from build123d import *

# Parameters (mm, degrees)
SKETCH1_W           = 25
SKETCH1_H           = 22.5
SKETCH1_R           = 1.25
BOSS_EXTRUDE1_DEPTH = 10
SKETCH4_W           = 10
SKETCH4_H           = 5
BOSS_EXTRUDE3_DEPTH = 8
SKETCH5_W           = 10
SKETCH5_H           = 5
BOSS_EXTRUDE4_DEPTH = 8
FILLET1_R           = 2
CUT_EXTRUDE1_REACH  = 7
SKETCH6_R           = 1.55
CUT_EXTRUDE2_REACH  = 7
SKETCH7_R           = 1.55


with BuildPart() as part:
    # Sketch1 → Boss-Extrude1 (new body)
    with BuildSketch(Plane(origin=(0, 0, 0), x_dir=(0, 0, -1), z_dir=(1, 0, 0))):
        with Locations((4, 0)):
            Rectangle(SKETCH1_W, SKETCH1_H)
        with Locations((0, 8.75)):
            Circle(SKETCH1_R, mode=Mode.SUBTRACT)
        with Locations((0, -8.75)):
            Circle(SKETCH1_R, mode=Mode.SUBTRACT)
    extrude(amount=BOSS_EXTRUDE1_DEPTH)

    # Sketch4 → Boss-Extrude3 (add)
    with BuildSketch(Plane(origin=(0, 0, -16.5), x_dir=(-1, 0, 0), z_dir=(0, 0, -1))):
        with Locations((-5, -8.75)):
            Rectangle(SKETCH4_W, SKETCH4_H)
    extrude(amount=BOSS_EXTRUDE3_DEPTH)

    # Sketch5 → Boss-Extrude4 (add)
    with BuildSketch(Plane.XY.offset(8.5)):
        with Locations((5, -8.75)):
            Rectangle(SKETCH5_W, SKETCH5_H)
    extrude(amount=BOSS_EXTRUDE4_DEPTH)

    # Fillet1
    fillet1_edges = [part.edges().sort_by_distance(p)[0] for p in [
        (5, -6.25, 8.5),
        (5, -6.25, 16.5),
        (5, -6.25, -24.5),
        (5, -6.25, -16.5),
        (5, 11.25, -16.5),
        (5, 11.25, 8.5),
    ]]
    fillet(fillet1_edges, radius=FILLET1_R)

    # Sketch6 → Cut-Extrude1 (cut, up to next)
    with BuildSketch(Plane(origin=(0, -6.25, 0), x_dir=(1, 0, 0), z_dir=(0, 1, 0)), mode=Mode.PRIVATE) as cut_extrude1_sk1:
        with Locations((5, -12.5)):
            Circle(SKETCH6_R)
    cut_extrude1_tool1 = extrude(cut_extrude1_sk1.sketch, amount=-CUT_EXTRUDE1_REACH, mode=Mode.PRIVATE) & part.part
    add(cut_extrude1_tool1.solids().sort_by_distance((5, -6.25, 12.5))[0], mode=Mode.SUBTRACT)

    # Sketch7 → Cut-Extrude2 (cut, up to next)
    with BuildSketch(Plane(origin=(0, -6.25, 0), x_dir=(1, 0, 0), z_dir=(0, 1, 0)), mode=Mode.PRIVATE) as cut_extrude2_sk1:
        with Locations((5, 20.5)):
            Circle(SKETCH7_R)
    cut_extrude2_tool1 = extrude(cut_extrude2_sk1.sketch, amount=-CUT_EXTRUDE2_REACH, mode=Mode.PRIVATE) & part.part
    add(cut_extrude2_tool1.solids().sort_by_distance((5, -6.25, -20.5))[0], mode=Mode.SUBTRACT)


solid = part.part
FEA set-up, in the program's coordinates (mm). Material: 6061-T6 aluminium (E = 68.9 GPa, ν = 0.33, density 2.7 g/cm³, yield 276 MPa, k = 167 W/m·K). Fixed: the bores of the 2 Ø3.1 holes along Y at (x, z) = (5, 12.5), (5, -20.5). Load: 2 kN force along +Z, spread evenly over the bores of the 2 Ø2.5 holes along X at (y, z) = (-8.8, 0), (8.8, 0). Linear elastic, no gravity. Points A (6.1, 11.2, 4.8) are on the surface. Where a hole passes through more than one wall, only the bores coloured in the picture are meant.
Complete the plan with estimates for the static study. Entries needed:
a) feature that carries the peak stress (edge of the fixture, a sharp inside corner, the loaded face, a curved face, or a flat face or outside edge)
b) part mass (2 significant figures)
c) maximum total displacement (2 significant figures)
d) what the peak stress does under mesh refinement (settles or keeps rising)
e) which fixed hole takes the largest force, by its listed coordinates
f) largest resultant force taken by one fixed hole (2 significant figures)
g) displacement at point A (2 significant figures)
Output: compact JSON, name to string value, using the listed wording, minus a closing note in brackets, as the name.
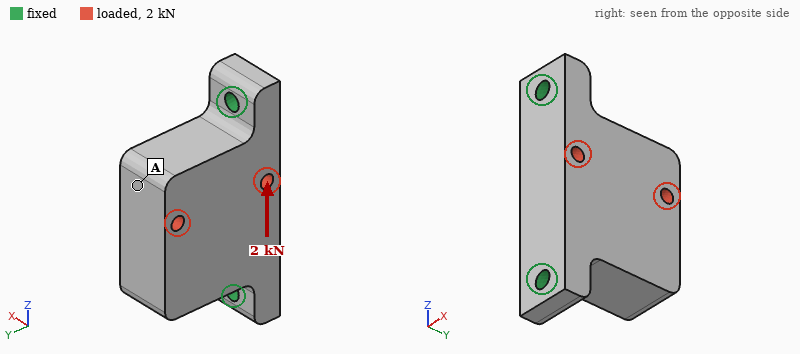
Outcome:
{"feature that carries the peak stress": "edge of the fixture", "part mass": "17 g", "maximum total displacement": "11 µm", "what the peak stress does under mesh refinement": "keeps rising", "which fixed hole takes the largest force, by its listed coordinates": "(5, 12.5)", "largest resultant force taken by one fixed hole": "1.2 kN", "displacement at point A": "11 µm"}
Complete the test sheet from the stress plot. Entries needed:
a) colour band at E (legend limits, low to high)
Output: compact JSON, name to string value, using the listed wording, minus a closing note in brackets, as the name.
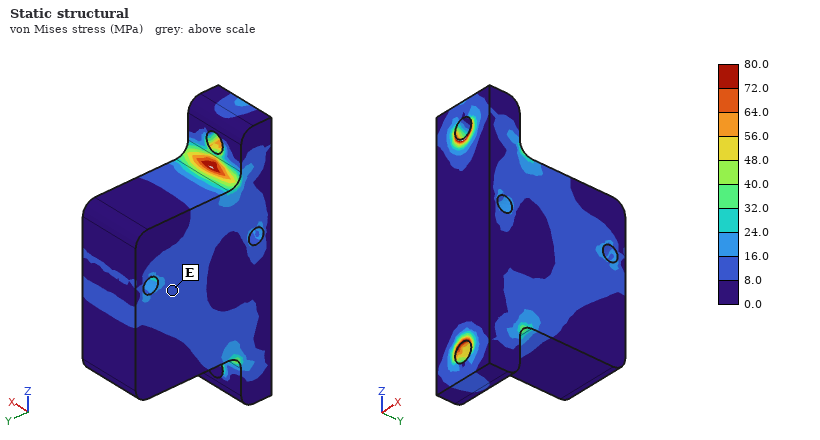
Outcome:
{"colour band at E": "8.0 to 16.0 MPa"}
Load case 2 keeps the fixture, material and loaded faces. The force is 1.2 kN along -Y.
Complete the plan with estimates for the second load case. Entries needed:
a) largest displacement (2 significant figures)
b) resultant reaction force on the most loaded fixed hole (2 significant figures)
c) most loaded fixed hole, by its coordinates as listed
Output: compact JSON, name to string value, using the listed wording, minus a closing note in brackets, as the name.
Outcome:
{"largest displacement": "7.1 µm", "resultant reaction force on the most loaded fixed hole": "830 N", "most loaded fixed hole, by its coordinates as listed": "(5, 12.5)"}
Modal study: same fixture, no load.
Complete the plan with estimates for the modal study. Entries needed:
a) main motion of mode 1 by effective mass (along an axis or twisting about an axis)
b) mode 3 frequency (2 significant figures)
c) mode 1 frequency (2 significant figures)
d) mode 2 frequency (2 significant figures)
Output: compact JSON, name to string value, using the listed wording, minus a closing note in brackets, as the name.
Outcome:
{"main motion of mode 1 by effective mass": "along X", "mode 3 frequency": "21 kHz", "mode 1 frequency": "6300 Hz", "mode 2 frequency": "20 kHz"}
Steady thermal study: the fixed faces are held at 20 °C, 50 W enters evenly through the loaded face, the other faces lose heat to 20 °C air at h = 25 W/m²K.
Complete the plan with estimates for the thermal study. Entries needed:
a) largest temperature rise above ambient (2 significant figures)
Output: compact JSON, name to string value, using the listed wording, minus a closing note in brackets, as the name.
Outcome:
{"largest temperature rise above ambient": "35 K"}
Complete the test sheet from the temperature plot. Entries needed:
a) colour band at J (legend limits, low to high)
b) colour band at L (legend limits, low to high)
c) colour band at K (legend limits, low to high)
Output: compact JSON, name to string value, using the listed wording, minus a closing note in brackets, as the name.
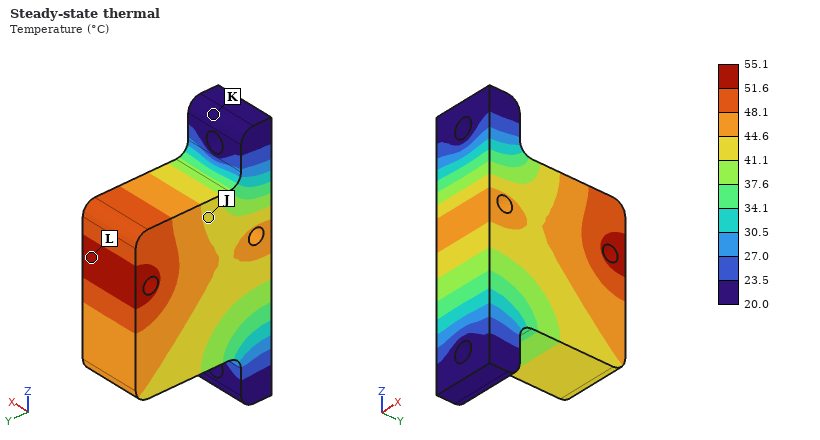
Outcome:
{"colour band at J": "41.1 to 44.6 °C", "colour band at L": "51.6 to 55.1 °C", "colour band at K": "20.0 to 23.5 °C"}
